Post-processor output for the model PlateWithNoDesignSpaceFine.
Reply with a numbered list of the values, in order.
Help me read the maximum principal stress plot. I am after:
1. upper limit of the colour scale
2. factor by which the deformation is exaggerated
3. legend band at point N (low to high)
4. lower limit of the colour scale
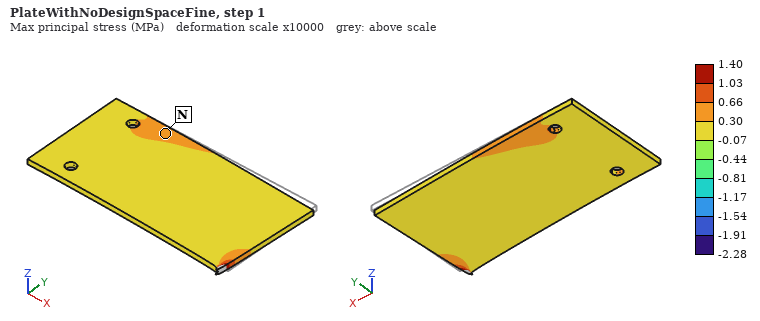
1. 1.40 MPa
2. 10000
3. 0.30 to 0.66 MPa
4. -2.28 MPa
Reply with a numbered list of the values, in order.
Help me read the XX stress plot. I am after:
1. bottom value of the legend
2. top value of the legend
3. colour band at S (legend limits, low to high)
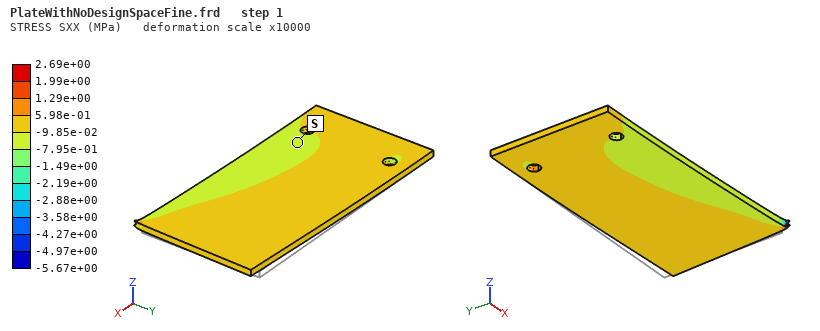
1. -5.67e+00 MPa
2. 2.69e+00 MPa
3. -7.95e-01 to -9.85e-02 MPa
